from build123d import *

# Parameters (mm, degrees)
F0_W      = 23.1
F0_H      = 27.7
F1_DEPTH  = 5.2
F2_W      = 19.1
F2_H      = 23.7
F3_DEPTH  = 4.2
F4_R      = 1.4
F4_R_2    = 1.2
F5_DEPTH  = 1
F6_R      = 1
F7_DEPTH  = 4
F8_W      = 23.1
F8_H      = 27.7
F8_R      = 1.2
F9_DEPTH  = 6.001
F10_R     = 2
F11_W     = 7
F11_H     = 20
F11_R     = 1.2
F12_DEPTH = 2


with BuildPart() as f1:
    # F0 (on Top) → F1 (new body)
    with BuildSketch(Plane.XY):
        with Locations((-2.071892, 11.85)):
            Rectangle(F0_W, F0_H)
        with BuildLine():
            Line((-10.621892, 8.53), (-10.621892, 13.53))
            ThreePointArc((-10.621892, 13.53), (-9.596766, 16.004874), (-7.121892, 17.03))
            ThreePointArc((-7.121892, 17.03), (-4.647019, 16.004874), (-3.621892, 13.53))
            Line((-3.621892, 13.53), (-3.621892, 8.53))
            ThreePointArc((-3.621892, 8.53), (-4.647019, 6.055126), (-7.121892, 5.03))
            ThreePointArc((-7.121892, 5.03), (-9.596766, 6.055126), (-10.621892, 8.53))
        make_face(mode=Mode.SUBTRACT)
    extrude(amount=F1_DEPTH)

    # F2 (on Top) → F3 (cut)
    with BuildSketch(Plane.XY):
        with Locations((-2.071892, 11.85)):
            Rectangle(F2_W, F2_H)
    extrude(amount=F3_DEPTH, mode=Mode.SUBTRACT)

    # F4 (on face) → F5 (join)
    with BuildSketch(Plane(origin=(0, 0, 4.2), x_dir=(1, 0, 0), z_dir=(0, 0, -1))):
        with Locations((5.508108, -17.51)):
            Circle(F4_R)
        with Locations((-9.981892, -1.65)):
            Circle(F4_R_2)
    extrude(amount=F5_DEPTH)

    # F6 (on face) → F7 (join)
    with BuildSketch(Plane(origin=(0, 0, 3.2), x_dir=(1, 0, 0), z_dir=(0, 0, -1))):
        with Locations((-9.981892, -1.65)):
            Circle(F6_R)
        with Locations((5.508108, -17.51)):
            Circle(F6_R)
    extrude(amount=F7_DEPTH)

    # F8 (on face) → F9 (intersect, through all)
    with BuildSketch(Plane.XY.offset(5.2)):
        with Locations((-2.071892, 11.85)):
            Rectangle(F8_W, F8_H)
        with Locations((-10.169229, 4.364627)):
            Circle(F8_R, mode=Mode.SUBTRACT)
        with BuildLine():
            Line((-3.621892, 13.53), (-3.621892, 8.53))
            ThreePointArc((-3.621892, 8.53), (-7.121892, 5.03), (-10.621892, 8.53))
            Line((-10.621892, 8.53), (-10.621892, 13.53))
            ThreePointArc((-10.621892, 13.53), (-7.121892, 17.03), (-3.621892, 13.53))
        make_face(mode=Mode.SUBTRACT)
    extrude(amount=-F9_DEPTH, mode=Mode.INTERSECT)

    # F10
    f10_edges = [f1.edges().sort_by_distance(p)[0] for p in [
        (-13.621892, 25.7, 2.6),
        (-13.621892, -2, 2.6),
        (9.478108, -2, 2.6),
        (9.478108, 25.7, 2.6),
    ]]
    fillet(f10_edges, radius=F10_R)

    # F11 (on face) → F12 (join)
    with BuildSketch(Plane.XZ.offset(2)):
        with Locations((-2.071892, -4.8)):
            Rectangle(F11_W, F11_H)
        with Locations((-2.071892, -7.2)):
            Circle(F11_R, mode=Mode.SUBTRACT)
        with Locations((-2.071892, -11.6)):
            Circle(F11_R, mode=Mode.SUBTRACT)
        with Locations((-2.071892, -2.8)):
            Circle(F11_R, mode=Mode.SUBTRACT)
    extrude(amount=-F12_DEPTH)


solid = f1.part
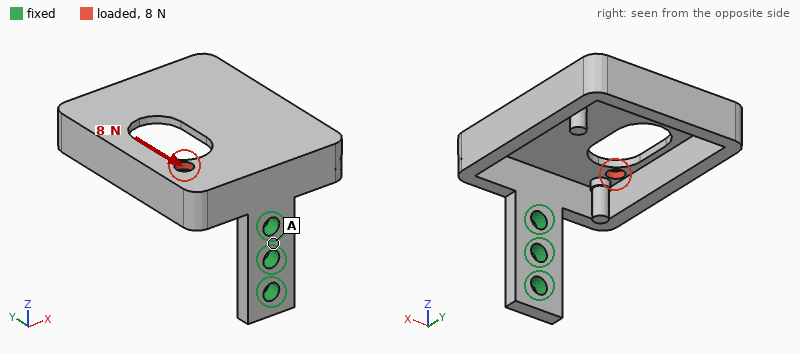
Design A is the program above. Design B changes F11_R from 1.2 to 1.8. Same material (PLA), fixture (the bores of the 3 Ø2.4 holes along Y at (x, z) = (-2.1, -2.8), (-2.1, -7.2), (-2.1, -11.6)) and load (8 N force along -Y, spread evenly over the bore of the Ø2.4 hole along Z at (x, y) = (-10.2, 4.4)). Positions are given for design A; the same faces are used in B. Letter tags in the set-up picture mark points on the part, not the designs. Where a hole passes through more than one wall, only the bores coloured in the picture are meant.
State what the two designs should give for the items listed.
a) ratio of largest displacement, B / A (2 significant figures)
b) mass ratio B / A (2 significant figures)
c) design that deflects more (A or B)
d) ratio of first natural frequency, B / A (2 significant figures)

0.80
0.98
A
1.1
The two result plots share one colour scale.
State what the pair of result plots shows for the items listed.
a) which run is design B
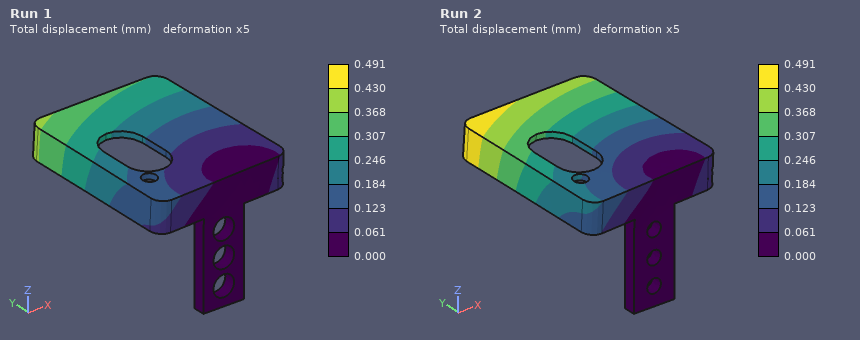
Run 1
